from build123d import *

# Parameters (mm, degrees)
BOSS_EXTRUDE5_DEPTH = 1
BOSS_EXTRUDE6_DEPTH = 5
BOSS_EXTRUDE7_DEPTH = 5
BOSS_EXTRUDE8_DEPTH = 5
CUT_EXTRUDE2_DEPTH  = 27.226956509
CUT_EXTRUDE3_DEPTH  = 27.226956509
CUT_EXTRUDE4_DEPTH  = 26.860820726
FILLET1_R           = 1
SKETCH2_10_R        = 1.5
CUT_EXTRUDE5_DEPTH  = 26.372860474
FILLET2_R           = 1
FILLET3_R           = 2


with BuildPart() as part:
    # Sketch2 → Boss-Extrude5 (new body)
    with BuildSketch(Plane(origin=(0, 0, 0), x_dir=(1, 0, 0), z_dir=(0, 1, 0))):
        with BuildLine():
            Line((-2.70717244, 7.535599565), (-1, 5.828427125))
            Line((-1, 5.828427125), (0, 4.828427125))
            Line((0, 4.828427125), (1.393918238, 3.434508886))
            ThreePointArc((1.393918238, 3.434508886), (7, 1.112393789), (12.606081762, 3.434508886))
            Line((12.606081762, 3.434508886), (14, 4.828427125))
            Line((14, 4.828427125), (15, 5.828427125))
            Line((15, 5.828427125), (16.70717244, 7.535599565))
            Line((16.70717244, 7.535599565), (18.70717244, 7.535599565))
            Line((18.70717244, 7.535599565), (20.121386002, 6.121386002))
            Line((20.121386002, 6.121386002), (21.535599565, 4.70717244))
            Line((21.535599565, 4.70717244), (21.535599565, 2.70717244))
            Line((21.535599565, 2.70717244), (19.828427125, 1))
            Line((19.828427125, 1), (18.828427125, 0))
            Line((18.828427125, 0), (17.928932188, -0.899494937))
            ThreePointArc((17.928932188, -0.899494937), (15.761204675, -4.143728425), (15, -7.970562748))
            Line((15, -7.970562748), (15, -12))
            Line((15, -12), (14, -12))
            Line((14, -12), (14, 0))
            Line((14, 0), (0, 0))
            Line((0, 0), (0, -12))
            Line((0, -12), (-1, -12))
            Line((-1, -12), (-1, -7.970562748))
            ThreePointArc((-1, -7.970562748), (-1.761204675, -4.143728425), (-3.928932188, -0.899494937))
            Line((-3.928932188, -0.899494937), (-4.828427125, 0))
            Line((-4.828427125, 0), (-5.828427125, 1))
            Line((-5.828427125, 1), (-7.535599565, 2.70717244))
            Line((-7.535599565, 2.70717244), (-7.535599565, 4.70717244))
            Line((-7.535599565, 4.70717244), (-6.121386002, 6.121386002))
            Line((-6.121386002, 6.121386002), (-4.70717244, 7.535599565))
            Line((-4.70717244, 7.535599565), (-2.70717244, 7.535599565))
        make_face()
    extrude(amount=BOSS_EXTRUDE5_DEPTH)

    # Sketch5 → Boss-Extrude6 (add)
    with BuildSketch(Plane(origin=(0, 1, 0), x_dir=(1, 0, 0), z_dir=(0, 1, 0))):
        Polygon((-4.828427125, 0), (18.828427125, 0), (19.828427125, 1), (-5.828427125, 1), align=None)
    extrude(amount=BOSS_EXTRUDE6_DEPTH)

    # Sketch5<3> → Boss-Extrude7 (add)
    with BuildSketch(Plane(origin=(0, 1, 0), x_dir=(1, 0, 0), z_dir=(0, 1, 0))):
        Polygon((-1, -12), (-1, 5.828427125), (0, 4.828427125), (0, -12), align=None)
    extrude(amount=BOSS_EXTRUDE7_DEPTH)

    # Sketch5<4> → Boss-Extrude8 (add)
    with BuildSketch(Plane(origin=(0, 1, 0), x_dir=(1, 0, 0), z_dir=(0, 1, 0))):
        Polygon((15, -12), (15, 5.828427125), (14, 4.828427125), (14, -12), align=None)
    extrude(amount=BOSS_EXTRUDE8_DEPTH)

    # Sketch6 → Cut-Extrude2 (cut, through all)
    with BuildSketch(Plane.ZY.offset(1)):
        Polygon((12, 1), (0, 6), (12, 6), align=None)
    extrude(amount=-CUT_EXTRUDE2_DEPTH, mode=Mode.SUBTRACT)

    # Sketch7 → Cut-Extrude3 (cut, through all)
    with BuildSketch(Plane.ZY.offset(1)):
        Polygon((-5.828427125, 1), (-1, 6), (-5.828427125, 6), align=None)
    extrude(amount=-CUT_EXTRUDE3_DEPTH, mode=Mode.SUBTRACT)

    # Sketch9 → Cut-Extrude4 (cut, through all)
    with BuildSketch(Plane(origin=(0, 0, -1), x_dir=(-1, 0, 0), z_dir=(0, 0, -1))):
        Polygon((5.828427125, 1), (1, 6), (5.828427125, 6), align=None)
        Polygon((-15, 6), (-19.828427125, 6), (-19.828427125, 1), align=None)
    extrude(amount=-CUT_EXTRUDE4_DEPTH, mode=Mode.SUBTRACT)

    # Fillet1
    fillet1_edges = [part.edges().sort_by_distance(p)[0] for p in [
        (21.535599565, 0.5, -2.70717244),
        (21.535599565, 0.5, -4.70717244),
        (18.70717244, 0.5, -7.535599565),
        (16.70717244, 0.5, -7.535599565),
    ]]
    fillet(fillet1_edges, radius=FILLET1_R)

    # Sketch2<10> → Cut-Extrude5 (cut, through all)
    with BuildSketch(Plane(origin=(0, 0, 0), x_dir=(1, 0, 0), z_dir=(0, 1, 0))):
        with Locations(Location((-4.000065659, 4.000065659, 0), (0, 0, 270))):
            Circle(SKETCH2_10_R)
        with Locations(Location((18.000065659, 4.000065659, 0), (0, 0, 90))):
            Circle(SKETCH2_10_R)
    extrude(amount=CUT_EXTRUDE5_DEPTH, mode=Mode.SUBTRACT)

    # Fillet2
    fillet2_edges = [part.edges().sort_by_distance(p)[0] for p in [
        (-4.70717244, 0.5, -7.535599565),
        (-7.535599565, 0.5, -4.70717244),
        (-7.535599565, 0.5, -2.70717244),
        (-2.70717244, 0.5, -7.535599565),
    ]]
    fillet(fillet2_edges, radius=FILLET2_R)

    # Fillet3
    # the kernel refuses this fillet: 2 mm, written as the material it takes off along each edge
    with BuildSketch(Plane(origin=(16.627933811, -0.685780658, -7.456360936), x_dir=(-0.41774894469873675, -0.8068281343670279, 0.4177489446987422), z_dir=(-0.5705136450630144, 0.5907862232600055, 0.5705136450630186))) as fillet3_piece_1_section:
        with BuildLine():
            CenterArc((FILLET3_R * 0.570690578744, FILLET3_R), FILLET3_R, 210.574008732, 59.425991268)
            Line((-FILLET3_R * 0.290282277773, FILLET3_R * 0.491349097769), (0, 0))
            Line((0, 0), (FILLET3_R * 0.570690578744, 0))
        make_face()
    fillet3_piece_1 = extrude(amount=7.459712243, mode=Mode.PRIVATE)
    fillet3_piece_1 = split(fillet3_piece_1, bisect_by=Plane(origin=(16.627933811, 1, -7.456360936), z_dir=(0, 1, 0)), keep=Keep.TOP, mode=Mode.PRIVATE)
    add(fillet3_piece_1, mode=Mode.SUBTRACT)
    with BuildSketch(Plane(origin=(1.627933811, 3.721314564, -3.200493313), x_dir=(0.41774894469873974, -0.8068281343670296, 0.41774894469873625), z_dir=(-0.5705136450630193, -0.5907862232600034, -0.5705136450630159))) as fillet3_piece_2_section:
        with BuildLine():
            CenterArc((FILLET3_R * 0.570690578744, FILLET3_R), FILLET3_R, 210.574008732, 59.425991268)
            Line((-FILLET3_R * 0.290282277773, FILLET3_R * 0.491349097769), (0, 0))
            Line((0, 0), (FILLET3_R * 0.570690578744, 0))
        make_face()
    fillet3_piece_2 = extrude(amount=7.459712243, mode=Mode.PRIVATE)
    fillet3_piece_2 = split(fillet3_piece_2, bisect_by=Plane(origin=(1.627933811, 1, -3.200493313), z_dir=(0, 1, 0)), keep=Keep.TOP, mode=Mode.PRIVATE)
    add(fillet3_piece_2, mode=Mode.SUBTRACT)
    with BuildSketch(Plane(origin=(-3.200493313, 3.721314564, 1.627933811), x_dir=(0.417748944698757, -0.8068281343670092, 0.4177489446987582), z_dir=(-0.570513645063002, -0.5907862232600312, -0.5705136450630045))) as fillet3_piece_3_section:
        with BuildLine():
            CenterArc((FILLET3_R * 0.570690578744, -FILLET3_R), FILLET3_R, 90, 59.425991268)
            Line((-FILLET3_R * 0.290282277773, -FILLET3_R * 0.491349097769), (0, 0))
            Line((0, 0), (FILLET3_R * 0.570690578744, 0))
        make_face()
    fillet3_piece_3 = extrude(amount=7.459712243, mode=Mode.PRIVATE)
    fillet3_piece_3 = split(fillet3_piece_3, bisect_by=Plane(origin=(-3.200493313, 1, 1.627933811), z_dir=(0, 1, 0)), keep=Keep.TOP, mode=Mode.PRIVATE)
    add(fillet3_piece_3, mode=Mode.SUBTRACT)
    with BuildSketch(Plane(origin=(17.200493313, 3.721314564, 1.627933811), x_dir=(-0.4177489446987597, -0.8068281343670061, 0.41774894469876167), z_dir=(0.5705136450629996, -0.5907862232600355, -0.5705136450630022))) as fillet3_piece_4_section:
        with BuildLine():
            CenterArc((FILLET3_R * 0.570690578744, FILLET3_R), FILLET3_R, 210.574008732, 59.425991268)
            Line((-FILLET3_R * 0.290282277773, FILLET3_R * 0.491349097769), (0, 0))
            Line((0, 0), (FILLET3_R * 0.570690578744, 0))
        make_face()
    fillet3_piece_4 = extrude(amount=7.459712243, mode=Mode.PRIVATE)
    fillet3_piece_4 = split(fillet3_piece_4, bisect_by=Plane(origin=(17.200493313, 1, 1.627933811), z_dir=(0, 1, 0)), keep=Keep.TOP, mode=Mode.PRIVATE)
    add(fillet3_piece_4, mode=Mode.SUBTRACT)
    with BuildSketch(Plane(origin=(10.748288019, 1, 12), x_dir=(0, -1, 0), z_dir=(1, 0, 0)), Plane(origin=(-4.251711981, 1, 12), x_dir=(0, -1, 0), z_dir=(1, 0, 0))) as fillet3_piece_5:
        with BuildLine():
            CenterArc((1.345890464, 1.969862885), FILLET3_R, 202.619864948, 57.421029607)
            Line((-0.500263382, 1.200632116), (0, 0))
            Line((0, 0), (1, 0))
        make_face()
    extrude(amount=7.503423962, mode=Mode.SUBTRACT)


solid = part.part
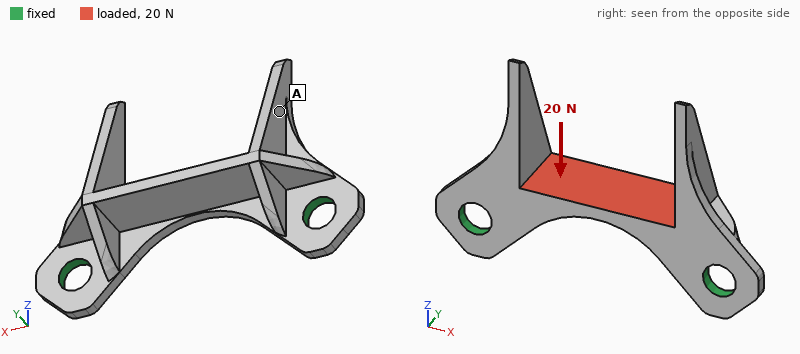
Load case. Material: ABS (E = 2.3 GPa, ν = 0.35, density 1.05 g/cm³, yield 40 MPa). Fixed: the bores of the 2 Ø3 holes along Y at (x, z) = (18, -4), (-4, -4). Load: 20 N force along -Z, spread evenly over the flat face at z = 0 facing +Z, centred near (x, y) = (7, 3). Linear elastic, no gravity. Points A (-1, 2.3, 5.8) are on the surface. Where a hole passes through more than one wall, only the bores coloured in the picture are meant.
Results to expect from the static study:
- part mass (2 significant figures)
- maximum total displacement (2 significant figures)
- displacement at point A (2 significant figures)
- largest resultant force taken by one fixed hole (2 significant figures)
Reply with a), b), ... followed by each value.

a) 0.35 g
b) 0.25 mm
c) 0.14 mm
d) 11 N
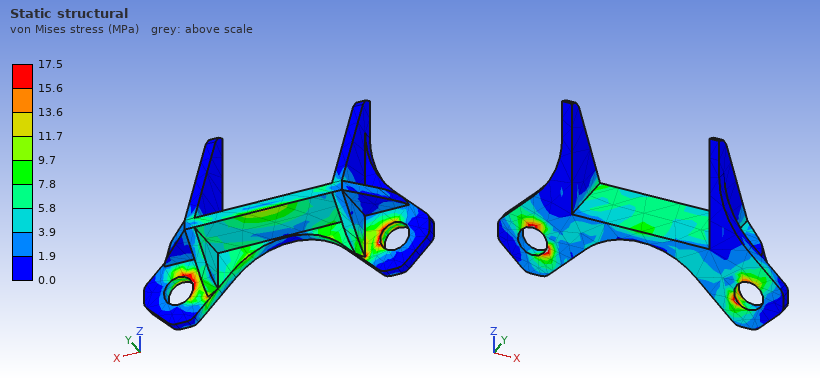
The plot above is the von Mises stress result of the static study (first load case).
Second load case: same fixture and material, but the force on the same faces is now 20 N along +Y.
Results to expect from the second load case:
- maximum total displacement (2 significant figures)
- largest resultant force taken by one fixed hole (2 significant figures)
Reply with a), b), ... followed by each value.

a) 0.28 mm
b) 14 N
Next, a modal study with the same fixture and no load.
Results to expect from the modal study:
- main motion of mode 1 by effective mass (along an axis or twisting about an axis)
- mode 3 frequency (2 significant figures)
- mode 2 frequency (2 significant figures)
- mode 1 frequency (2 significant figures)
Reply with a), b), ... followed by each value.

a) along Y
b) 4400 Hz
c) 3900 Hz
d) 3000 Hz
